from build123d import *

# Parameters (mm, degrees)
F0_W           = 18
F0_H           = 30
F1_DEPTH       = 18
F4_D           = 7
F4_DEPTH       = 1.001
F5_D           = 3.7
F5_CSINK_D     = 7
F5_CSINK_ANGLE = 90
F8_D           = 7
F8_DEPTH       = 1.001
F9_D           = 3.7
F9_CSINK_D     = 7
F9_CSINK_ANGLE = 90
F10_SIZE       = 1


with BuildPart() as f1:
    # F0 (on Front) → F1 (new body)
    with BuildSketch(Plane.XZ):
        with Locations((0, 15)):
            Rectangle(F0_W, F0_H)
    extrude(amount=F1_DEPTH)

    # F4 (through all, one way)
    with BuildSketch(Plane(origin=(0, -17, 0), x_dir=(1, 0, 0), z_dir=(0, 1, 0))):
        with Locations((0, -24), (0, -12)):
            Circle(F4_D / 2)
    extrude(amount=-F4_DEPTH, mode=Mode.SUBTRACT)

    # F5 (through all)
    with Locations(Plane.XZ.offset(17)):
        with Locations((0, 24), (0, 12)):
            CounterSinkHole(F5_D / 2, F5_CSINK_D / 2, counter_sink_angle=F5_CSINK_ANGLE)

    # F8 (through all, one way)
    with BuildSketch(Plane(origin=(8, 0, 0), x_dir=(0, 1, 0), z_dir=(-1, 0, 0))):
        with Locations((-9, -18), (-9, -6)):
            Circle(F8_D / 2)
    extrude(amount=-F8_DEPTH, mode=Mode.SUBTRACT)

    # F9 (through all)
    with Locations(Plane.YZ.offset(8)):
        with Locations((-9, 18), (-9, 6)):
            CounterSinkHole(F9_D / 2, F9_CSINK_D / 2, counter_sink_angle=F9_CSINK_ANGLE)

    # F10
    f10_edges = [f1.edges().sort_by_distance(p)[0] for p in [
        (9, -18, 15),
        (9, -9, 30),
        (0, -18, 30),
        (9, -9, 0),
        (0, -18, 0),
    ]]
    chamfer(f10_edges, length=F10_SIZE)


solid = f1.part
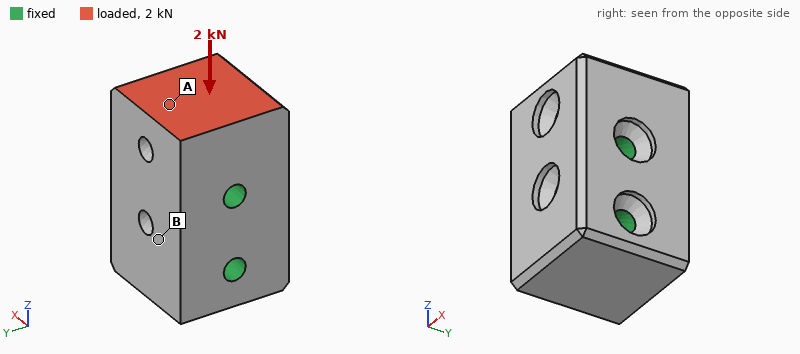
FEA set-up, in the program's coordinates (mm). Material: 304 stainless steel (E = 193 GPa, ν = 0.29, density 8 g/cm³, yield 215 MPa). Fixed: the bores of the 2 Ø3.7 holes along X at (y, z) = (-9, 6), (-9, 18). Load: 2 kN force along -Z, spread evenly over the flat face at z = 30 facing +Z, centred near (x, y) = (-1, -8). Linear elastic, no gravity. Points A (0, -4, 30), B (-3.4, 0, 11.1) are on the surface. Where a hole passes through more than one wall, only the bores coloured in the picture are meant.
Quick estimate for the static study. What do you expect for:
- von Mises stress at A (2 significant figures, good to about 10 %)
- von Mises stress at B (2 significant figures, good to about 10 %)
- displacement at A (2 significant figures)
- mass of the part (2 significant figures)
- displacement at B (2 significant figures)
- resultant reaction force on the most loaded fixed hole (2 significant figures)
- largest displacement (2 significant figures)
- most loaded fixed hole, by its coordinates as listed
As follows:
5.9 MPa
2.3 MPa
0.74 µm
70 g
0.13 µm
1.6 kN
0.82 µm
(-9, 18)
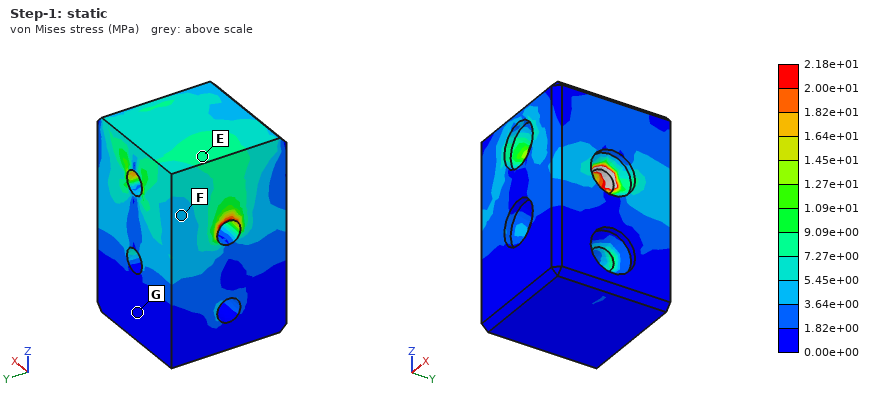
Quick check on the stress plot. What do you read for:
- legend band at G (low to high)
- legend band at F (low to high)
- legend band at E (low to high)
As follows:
0.00e+00 to 1.82e+00 MPa
3.64e+00 to 5.45e+00 MPa
7.27e+00 to 9.09e+00 MPa
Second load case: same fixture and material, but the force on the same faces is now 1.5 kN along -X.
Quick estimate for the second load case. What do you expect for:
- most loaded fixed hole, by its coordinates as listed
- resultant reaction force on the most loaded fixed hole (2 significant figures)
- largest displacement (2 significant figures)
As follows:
(-9, 18)
1.7 kN
2.8 µm
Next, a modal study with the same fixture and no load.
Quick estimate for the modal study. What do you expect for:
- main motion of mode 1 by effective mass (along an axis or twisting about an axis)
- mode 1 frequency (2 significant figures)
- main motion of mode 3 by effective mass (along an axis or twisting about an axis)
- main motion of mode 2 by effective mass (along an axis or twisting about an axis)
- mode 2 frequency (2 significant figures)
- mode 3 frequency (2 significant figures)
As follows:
along Y
33 kHz
twisting about Z
along X
38 kHz
45 kHz
